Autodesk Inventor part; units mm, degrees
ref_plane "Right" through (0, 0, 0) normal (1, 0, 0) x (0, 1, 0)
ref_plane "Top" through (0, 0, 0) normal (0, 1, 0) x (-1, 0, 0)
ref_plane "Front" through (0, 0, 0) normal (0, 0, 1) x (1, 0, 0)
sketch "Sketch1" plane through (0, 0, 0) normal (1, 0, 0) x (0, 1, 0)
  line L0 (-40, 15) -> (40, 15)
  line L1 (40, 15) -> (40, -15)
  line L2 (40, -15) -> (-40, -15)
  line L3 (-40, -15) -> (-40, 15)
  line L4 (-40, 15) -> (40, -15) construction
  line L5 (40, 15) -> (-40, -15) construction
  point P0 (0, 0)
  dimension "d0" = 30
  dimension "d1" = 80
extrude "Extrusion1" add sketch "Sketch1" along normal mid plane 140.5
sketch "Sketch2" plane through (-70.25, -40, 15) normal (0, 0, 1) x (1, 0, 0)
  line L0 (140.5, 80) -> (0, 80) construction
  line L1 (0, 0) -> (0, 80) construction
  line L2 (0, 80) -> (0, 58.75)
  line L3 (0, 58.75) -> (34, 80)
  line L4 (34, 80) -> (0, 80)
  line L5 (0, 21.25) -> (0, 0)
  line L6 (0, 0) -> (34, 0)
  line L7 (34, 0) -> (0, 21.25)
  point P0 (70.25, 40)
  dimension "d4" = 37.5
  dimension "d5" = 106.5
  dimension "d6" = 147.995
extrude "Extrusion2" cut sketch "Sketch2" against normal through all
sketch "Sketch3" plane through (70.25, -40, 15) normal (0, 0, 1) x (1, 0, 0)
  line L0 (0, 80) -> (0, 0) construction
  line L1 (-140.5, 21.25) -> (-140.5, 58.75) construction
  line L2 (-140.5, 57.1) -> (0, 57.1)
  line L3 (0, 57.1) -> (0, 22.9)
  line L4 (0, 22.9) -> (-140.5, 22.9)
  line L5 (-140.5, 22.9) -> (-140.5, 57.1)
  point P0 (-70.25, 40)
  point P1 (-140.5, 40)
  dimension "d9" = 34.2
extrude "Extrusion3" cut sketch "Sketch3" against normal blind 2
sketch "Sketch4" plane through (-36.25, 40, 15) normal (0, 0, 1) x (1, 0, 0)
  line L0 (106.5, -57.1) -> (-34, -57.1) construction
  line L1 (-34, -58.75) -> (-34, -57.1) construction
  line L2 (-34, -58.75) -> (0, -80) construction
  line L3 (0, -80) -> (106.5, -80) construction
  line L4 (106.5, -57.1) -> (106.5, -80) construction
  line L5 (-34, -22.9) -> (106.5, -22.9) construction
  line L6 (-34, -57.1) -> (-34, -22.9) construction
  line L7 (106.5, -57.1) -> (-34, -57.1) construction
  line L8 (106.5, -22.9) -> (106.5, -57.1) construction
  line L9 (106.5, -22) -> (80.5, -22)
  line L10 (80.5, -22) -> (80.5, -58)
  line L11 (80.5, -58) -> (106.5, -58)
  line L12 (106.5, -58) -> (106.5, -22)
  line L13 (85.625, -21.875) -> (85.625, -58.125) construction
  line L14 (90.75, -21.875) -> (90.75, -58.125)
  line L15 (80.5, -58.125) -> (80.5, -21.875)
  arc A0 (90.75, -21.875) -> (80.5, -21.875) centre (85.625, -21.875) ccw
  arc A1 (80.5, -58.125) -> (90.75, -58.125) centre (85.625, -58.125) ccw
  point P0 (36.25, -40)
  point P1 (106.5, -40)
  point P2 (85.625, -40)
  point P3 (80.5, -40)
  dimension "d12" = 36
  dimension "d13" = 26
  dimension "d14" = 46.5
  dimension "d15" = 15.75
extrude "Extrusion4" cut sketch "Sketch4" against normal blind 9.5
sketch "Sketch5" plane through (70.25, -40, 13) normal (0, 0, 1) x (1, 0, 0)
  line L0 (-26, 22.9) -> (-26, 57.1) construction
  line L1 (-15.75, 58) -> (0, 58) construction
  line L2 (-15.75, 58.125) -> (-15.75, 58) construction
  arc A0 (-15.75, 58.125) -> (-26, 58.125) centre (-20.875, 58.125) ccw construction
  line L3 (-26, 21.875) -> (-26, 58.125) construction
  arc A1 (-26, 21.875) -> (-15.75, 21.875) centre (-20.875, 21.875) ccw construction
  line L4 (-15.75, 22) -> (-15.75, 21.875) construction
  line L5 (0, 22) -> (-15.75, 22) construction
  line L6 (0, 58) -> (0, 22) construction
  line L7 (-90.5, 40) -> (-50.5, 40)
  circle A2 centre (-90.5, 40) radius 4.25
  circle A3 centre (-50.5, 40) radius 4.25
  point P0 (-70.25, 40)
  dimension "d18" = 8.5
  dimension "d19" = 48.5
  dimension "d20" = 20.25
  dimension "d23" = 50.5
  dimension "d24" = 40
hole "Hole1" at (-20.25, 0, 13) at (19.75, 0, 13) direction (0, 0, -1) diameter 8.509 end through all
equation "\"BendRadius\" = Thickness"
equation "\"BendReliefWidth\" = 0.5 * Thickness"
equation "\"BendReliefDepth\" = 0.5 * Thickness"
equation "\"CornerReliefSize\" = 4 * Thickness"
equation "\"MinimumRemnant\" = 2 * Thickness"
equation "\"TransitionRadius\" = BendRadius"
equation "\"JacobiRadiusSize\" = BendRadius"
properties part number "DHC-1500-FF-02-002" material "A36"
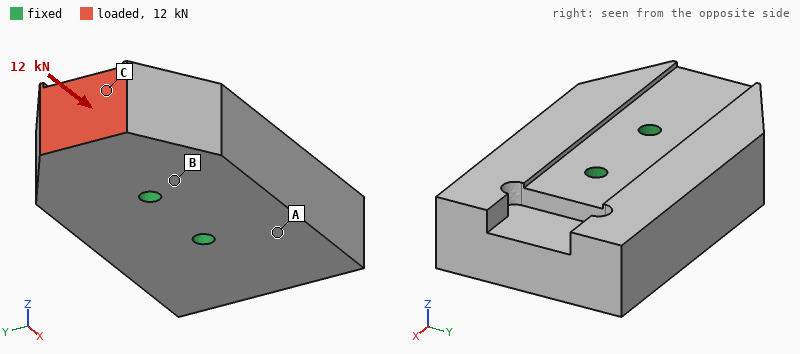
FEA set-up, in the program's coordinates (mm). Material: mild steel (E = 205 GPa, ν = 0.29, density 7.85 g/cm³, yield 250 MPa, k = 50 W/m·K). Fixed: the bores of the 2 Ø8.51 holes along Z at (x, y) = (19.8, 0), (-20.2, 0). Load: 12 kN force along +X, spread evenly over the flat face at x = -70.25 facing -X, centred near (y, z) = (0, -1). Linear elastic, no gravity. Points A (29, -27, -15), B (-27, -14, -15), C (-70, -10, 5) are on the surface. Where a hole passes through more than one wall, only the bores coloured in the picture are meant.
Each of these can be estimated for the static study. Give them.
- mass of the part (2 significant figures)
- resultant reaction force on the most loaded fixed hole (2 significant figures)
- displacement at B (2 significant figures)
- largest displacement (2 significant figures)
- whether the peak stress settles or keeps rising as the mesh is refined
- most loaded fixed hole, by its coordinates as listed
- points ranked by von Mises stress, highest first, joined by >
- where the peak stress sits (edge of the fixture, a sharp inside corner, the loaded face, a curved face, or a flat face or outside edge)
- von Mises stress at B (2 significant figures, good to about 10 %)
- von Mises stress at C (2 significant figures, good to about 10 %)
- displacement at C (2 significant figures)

2.3 kg
8.8 kN
0.78 µm
2.8 µm
keeps rising
(-20.2, 0)
C > B > A
edge of the fixture
4.9 MPa
9.3 MPa
2.5 µm
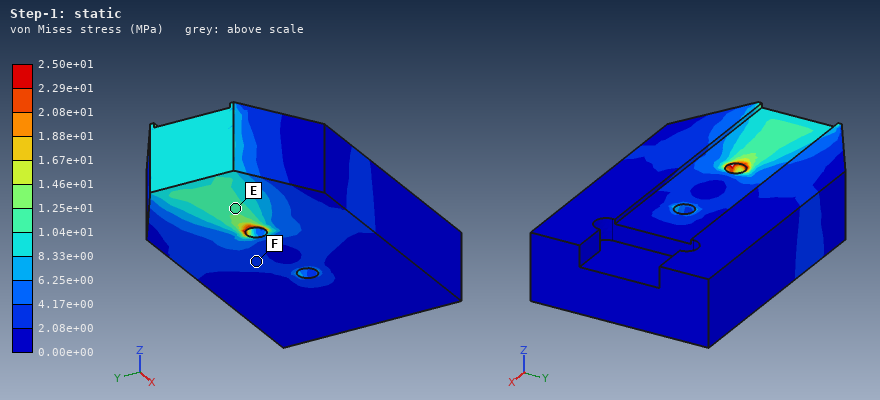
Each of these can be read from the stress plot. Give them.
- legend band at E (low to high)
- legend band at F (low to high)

1.04e+01 to 1.25e+01 MPa
2.08e+00 to 4.17e+00 MPa
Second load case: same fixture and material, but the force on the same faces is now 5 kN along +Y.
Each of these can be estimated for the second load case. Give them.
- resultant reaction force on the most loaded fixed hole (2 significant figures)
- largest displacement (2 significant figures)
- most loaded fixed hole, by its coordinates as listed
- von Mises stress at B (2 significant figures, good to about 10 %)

10 kN
6.4 µm
(-20.2, 0)
6.8 MPa
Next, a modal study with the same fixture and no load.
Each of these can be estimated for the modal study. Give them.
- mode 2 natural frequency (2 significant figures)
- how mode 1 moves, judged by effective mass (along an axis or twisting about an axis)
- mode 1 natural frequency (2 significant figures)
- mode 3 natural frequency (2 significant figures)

6400 Hz
along Z
5900 Hz
6400 Hz
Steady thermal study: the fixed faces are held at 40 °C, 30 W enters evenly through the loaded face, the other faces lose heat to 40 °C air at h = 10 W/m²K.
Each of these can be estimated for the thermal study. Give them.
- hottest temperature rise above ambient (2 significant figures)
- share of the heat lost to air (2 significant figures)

21 K
4.1 %
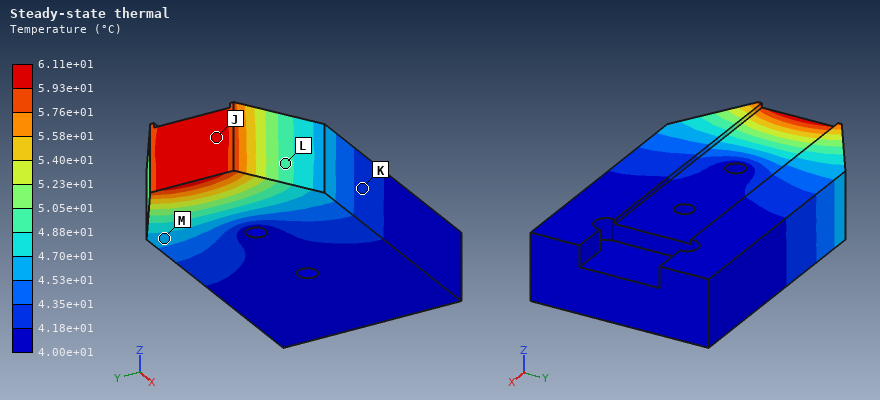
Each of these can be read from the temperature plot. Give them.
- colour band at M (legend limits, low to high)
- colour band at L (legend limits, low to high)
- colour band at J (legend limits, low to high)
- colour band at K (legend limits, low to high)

4.53e+01 to 4.70e+01 °C
4.88e+01 to 5.05e+01 °C
5.93e+01 to 6.11e+01 °C
4.18e+01 to 4.35e+01 °C
